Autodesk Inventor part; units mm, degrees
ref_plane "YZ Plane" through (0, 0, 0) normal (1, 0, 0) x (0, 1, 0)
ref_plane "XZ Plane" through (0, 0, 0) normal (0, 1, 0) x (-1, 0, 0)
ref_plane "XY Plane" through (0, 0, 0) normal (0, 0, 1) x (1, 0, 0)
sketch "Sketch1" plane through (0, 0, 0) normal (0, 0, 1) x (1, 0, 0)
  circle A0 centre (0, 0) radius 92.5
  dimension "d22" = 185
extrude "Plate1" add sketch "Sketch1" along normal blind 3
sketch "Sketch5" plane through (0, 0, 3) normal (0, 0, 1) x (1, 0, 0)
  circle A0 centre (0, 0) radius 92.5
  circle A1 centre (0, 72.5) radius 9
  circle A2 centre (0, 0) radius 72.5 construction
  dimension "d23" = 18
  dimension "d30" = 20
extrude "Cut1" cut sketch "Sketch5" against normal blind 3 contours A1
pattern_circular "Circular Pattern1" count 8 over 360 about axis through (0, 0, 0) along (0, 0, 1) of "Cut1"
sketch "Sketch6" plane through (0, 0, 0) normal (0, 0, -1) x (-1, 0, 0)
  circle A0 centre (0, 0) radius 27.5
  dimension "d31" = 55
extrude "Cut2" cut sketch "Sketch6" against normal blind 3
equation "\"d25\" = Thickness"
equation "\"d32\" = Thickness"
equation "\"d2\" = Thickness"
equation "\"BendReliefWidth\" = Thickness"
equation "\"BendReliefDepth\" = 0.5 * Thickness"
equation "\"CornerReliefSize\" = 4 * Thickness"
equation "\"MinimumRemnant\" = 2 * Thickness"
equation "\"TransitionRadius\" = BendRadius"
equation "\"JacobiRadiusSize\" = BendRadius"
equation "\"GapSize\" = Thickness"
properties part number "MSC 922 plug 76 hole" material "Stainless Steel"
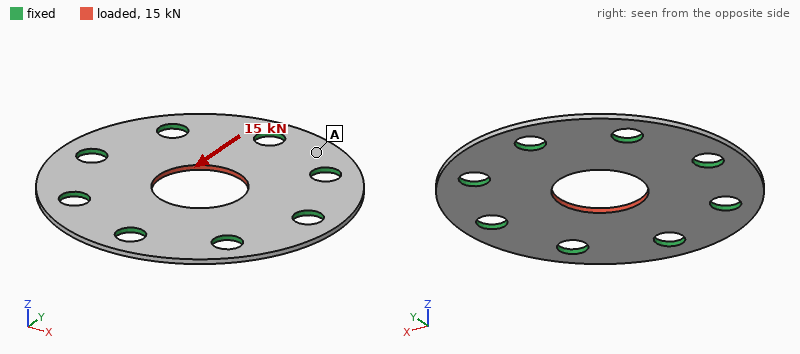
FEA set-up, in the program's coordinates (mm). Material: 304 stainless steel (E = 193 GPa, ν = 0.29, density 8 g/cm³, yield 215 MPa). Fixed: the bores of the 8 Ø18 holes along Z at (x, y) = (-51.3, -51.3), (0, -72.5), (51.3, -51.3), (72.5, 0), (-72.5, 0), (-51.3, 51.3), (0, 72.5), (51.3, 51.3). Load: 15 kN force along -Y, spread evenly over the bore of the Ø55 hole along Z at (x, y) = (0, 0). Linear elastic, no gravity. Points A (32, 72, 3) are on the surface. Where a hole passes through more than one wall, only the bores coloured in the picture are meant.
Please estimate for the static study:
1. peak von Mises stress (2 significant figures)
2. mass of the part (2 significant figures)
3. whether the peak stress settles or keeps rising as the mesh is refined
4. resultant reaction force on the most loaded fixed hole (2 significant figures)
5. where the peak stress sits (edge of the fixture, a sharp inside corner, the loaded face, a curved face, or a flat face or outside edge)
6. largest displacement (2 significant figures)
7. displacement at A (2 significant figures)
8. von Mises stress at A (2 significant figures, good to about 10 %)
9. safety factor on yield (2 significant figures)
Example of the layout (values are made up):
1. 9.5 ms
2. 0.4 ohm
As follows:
1. 50 MPa
2. 540 g
3. settles
4. 3.1 kN
5. the loaded face
6. 6.3 µm
7. 1.3 µm
8. 5.3 MPa
9. 4.3
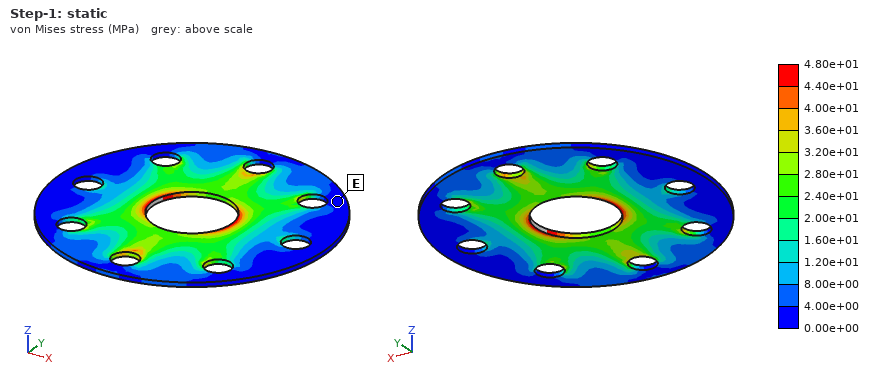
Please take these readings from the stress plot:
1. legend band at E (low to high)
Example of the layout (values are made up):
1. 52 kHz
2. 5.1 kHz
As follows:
1. 0.00e+00 to 4.00e+00 MPa
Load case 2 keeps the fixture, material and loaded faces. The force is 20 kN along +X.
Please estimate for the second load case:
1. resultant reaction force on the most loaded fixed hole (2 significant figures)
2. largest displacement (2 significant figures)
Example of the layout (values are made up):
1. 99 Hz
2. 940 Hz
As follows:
1. 4.1 kN
2. 8.4 µm
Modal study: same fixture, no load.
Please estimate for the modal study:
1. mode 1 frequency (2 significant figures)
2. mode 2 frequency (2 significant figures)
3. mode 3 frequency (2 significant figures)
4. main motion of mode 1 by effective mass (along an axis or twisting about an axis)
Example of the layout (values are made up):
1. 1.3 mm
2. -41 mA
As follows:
1. 2200 Hz
2. 3000 Hz
3. 3000 Hz
4. along Z
